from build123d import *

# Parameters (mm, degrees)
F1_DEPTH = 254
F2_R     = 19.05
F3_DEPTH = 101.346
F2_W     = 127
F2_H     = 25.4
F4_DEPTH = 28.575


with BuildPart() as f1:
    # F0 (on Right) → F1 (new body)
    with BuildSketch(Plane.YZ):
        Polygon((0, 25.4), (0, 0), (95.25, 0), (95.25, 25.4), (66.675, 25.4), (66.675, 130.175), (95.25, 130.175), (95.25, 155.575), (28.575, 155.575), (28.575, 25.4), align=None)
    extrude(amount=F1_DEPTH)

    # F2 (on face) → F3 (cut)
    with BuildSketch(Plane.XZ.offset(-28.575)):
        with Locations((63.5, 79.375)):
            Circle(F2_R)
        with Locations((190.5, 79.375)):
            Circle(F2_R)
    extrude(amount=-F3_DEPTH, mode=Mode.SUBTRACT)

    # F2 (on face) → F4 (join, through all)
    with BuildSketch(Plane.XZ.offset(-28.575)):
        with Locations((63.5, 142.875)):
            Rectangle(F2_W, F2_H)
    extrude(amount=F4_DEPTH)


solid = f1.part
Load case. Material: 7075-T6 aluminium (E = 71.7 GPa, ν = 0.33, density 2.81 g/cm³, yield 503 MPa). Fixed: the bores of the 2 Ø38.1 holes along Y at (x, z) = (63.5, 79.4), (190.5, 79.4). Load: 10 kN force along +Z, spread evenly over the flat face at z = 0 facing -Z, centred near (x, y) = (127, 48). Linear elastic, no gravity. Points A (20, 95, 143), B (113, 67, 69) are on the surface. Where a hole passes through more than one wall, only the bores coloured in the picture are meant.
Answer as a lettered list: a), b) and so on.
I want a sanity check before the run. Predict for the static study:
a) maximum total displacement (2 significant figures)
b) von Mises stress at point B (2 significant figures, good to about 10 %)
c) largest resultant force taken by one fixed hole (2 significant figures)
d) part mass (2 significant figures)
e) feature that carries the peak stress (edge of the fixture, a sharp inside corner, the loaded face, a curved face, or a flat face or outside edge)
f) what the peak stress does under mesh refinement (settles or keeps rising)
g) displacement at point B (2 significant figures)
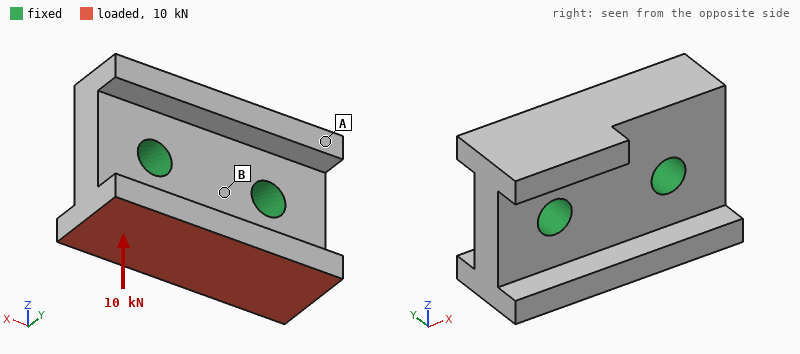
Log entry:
a) 2.7 µm
b) 0.46 MPa
c) 5.0 kN
d) 5.8 kg
e) edge of the fixture
f) keeps rising
g) 0.51 µm
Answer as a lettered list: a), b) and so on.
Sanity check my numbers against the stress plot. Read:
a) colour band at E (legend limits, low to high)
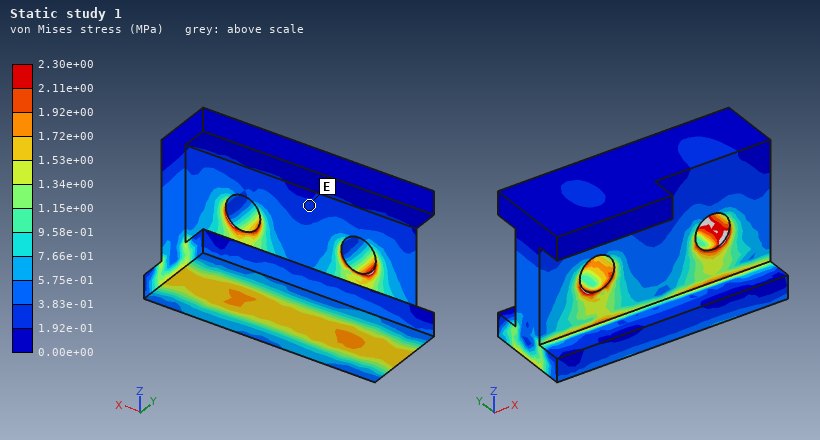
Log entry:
a) 1.92e-01 to 3.83e-01 MPa
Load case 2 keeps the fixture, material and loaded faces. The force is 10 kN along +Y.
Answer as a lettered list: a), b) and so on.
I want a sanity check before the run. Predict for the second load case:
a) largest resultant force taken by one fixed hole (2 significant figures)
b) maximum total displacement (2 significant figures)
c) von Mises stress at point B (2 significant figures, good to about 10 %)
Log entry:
a) 5.0 kN
b) 25 µm
c) 4.4 MPa
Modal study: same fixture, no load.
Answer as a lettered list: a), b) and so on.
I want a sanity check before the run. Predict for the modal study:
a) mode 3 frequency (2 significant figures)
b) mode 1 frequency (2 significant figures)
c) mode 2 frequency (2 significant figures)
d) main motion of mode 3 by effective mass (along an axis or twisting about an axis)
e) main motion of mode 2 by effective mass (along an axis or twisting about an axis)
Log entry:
a) 3500 Hz
b) 2900 Hz
c) 3400 Hz
d) along Y
e) along Y
